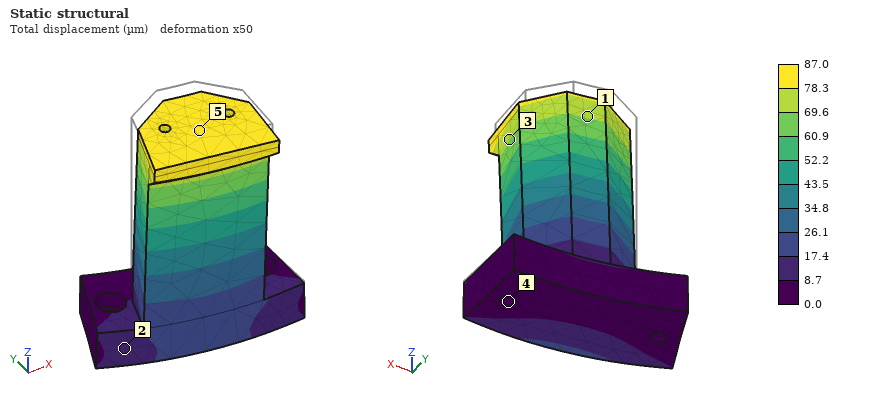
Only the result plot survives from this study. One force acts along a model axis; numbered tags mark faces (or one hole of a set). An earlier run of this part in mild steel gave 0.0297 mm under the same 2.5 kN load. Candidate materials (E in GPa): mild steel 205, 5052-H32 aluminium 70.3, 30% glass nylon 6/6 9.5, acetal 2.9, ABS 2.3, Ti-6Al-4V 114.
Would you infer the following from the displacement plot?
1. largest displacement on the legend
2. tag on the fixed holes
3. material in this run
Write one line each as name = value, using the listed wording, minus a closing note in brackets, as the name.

largest displacement on the legend = 87.0 µm
tag on the fixed holes = 4
material in this run = 5052-H32 aluminium
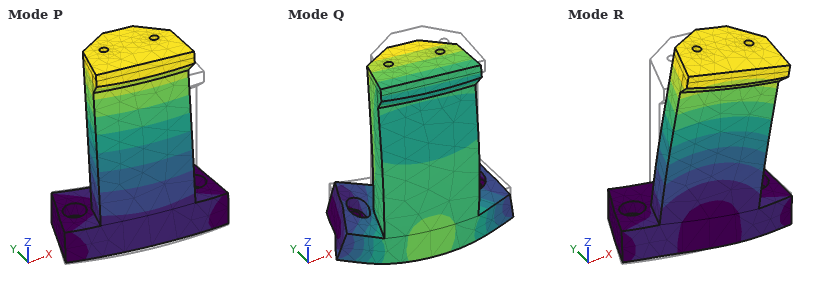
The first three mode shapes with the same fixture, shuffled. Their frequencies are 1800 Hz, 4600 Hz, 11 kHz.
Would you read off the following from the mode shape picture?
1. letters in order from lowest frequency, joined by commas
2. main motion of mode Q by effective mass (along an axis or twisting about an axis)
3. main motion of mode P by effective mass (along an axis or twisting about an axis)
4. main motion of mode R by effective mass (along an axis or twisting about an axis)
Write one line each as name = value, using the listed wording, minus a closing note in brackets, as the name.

letters in order from lowest frequency, joined by commas = P, R, Q
main motion of mode Q by effective mass = along Z
main motion of mode P by effective mass = along Y
main motion of mode R by effective mass = along X
